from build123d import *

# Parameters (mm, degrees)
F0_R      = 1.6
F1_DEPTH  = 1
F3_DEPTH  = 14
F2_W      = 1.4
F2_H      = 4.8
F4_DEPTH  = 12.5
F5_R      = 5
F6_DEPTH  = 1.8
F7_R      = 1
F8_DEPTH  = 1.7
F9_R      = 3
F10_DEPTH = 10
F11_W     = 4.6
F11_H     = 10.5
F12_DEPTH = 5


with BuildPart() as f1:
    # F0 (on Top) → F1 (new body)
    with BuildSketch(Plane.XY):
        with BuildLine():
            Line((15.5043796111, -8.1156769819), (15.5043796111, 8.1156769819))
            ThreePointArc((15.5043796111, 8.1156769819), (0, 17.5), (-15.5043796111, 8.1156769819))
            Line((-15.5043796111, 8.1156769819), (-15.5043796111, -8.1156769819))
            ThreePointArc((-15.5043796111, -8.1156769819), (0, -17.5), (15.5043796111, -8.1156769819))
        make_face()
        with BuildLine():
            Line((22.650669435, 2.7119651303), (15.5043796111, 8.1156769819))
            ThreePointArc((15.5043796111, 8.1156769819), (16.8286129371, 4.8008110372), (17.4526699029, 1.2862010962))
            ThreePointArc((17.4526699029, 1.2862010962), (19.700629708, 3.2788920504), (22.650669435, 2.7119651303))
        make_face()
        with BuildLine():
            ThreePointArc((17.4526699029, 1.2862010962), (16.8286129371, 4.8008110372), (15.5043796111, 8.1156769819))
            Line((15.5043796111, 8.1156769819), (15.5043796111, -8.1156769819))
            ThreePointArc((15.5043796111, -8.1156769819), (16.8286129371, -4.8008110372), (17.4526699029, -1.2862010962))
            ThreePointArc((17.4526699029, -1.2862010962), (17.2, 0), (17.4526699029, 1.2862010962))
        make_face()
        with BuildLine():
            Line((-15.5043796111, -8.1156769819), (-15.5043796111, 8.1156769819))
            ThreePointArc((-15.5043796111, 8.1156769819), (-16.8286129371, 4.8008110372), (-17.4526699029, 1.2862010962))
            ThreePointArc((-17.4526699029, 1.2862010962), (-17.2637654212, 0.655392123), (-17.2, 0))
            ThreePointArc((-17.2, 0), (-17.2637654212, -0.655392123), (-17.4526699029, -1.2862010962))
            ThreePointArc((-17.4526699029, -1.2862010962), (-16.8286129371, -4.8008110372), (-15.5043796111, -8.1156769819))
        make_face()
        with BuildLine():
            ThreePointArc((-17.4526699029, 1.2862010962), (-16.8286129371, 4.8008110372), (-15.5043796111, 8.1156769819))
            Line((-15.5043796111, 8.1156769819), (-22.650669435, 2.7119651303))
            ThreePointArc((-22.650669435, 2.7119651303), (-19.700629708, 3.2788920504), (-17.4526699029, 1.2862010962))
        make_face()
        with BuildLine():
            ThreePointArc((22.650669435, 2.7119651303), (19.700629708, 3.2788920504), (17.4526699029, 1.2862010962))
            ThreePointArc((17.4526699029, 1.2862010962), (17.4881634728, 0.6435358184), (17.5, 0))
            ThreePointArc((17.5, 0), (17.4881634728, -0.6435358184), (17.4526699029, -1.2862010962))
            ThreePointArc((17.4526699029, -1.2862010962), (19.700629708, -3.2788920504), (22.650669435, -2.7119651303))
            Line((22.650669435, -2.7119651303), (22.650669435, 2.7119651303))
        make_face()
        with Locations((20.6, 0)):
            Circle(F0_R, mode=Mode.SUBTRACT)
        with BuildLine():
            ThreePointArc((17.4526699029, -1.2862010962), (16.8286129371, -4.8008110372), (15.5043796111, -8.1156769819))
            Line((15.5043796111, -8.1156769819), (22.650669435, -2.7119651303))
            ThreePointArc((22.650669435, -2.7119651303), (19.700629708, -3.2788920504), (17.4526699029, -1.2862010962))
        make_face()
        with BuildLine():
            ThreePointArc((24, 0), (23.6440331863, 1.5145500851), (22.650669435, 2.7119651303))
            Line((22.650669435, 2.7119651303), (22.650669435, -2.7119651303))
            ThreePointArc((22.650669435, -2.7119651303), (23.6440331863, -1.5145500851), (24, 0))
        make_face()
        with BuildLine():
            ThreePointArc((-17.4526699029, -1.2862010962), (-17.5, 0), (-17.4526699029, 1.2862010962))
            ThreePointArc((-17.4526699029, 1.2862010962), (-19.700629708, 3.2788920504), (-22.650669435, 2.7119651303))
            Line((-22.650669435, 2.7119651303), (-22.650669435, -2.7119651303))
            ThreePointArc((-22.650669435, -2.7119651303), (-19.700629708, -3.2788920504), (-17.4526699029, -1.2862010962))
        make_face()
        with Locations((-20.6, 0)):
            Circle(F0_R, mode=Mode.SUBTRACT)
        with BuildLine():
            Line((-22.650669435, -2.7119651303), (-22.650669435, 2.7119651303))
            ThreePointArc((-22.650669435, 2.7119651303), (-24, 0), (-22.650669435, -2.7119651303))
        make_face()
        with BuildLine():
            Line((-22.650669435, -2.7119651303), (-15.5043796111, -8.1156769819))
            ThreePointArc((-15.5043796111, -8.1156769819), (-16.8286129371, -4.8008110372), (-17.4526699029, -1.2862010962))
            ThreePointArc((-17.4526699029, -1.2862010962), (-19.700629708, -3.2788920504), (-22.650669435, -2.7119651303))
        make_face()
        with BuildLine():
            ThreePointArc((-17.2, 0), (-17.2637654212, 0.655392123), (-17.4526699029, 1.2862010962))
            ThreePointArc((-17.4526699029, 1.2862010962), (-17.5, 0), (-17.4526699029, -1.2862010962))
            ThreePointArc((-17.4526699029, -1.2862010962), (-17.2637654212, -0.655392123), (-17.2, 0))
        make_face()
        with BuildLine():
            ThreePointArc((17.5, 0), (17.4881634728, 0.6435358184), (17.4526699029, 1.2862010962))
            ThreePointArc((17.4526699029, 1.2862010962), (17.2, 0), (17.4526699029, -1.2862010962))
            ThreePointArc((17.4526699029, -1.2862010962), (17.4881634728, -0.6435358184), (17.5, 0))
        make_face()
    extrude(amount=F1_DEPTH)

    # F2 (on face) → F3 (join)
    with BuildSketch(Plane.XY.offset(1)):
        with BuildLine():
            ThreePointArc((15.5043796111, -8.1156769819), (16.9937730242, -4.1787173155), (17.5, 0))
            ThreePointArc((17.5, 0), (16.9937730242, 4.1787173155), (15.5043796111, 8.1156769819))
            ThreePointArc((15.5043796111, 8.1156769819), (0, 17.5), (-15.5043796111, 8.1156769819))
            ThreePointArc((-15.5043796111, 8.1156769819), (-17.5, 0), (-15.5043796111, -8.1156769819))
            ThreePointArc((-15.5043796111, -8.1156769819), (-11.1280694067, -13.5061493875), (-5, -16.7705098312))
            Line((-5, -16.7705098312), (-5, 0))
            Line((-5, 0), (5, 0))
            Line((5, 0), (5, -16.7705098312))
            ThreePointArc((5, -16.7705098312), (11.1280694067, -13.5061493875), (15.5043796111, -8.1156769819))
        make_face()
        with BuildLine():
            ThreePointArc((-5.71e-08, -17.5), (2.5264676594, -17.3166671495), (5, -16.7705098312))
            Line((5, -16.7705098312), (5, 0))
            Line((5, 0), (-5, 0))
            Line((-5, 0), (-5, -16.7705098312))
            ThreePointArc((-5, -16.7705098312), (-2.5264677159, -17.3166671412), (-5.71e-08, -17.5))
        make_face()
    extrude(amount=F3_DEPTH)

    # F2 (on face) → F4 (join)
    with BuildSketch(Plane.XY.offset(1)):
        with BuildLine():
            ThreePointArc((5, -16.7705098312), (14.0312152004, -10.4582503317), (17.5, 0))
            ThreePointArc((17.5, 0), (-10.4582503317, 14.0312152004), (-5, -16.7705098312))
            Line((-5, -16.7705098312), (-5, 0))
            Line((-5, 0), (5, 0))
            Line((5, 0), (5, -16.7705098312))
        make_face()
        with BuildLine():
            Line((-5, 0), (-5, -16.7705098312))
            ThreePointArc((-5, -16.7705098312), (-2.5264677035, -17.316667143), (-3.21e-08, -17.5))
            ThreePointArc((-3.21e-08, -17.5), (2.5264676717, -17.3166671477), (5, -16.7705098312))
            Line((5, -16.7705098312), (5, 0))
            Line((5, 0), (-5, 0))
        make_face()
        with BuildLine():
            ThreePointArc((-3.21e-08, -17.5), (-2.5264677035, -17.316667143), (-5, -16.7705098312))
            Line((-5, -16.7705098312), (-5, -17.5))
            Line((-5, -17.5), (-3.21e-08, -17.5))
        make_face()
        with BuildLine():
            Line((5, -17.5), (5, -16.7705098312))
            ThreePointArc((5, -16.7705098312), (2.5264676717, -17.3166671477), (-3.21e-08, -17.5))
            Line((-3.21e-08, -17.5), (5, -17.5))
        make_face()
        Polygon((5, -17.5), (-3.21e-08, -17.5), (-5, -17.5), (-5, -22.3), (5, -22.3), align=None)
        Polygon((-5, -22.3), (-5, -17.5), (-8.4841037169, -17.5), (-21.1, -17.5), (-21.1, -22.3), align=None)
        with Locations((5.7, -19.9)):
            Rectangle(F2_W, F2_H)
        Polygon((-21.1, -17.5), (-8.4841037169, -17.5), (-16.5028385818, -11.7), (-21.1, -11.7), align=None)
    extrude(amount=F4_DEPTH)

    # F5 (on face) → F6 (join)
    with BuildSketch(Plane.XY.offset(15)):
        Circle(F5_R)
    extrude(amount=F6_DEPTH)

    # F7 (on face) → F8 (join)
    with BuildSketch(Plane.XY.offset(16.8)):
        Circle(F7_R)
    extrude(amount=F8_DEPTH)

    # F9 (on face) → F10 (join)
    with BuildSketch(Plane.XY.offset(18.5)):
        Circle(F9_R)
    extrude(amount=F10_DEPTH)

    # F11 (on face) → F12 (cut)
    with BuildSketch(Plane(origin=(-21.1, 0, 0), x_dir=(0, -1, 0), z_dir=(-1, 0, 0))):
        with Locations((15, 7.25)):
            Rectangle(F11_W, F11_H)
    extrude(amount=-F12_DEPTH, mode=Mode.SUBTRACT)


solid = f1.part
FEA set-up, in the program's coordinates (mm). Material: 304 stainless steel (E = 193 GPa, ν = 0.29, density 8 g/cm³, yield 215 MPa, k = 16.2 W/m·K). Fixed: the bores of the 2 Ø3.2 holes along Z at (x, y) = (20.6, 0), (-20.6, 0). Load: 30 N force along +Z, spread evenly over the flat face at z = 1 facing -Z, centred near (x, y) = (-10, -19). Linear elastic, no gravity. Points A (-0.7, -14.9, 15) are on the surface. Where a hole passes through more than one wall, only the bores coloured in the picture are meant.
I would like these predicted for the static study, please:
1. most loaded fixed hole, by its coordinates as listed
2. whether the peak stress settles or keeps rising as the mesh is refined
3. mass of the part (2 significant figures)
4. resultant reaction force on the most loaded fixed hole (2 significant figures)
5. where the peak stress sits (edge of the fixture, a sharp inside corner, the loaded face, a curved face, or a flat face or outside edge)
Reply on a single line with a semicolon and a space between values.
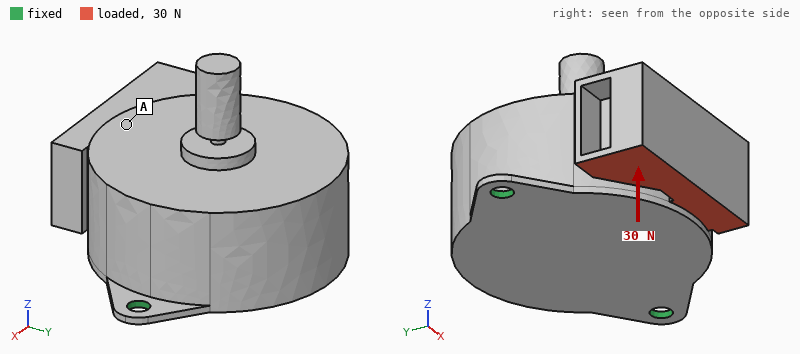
(-20.6, 0); keeps rising; 140 g; 25 N; edge of the fixture
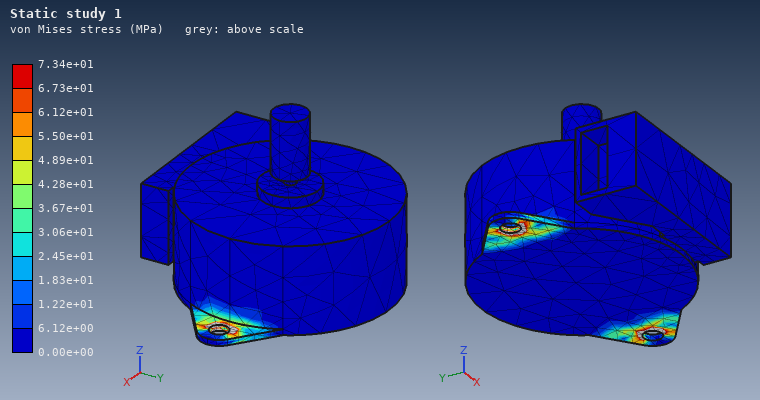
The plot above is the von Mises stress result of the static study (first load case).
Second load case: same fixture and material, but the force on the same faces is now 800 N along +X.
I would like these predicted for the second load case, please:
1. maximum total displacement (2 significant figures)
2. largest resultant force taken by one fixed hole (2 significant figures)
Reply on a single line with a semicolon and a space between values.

12 µm; 550 N
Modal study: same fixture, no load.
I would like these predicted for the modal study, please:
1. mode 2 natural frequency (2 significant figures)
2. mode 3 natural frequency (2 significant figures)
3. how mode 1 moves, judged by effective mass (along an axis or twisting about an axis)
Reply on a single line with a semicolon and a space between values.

3700 Hz; 3900 Hz; along Y
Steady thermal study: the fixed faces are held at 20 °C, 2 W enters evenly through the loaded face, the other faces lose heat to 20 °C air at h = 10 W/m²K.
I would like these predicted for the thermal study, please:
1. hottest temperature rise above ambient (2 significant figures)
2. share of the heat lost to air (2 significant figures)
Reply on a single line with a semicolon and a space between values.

39 K; 45 %
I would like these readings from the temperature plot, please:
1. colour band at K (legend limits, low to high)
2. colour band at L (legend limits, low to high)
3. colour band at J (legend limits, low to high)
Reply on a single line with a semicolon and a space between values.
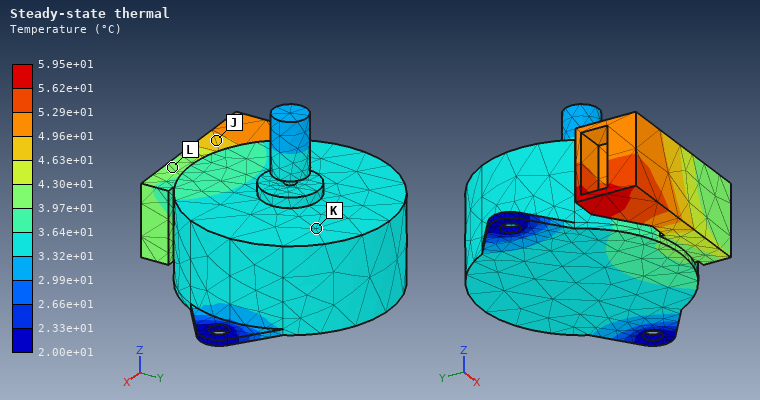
3.32e+01 to 3.64e+01 °C; 3.97e+01 to 4.30e+01 °C; 4.63e+01 to 4.96e+01 °C
